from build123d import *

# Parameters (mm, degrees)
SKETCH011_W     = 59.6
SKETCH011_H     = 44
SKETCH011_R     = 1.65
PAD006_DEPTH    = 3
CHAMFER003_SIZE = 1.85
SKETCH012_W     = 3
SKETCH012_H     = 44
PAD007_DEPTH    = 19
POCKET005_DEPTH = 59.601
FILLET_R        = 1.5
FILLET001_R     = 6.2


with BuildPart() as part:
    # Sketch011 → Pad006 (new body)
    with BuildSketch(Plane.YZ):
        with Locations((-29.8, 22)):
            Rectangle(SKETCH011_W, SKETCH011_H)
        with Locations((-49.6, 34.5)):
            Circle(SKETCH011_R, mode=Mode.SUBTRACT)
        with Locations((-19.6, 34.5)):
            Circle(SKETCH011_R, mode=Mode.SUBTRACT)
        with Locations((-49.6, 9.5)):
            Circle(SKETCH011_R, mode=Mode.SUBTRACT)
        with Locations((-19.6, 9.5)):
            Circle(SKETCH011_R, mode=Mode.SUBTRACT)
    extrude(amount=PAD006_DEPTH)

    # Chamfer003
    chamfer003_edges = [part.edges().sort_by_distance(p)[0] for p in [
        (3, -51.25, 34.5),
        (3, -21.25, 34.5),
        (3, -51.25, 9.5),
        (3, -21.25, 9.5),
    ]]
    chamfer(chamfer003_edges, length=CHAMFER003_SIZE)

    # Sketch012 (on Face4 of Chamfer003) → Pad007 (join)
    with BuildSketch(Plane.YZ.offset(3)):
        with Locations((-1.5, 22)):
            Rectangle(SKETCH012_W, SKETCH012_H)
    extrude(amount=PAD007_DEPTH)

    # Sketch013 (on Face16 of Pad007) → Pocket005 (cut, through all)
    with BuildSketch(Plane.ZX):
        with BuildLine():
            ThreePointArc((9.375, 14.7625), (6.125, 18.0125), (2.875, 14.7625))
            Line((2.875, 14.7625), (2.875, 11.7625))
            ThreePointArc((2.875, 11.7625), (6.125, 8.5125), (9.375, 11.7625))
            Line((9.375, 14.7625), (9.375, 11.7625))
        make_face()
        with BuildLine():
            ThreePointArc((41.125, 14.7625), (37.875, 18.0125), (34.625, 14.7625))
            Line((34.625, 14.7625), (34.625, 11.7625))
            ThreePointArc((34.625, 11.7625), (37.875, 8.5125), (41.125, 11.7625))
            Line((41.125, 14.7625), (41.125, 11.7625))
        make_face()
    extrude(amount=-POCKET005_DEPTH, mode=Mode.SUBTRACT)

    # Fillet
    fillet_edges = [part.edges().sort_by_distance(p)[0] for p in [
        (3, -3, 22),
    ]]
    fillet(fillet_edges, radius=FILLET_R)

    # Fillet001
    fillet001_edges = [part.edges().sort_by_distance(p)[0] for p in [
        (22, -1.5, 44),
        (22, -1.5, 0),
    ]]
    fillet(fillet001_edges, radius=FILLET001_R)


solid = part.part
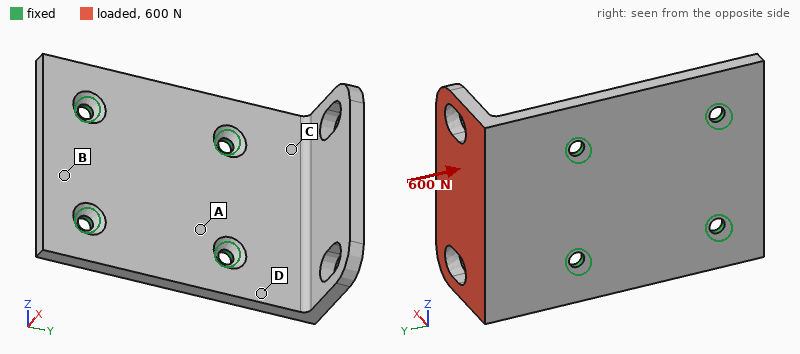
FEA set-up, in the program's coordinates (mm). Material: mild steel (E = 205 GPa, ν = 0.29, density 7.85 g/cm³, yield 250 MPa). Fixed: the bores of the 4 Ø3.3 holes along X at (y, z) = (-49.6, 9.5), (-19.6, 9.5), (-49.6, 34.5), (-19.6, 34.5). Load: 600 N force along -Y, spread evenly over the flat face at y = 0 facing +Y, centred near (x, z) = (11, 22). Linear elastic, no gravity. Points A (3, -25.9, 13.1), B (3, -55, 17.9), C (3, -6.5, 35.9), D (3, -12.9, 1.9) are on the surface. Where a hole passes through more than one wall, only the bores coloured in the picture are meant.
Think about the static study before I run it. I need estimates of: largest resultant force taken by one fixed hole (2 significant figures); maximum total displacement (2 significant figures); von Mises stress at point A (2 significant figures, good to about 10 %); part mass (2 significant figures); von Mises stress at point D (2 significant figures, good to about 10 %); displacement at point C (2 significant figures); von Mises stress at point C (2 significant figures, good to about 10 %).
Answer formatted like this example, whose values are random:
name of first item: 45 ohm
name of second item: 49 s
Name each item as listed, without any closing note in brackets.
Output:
largest resultant force taken by one fixed hole: 350 N
maximum total displacement: 0.16 mm
von Mises stress at point A: 27 MPa
part mass: 77 g
von Mises stress at point D: 90 MPa
displacement at point C: 0.038 mm
von Mises stress at point C: 75 MPa
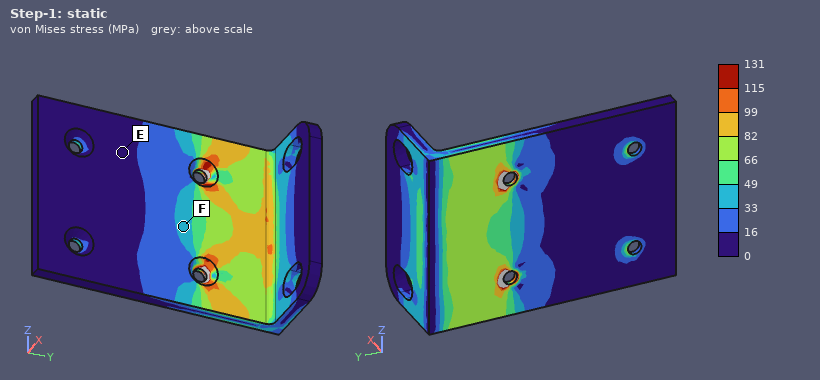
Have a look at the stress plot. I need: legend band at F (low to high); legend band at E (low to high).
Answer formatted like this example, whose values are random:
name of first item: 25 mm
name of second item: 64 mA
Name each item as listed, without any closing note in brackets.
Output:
legend band at F: 33 to 49 MPa
legend band at E: 0 to 16 MPa
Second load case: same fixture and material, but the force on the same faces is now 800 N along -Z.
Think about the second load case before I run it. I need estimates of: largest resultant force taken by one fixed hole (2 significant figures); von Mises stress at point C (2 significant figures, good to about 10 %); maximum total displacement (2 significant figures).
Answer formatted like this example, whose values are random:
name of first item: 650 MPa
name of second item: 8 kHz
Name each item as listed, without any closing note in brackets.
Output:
largest resultant force taken by one fixed hole: 780 N
von Mises stress at point C: 47 MPa
maximum total displacement: 53 µm
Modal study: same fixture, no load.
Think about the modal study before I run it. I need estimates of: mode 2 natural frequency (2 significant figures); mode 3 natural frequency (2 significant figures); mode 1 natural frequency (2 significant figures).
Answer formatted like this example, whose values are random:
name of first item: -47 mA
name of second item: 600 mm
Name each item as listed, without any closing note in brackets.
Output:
mode 2 natural frequency: 3800 Hz
mode 3 natural frequency: 6000 Hz
mode 1 natural frequency: 2000 Hz
